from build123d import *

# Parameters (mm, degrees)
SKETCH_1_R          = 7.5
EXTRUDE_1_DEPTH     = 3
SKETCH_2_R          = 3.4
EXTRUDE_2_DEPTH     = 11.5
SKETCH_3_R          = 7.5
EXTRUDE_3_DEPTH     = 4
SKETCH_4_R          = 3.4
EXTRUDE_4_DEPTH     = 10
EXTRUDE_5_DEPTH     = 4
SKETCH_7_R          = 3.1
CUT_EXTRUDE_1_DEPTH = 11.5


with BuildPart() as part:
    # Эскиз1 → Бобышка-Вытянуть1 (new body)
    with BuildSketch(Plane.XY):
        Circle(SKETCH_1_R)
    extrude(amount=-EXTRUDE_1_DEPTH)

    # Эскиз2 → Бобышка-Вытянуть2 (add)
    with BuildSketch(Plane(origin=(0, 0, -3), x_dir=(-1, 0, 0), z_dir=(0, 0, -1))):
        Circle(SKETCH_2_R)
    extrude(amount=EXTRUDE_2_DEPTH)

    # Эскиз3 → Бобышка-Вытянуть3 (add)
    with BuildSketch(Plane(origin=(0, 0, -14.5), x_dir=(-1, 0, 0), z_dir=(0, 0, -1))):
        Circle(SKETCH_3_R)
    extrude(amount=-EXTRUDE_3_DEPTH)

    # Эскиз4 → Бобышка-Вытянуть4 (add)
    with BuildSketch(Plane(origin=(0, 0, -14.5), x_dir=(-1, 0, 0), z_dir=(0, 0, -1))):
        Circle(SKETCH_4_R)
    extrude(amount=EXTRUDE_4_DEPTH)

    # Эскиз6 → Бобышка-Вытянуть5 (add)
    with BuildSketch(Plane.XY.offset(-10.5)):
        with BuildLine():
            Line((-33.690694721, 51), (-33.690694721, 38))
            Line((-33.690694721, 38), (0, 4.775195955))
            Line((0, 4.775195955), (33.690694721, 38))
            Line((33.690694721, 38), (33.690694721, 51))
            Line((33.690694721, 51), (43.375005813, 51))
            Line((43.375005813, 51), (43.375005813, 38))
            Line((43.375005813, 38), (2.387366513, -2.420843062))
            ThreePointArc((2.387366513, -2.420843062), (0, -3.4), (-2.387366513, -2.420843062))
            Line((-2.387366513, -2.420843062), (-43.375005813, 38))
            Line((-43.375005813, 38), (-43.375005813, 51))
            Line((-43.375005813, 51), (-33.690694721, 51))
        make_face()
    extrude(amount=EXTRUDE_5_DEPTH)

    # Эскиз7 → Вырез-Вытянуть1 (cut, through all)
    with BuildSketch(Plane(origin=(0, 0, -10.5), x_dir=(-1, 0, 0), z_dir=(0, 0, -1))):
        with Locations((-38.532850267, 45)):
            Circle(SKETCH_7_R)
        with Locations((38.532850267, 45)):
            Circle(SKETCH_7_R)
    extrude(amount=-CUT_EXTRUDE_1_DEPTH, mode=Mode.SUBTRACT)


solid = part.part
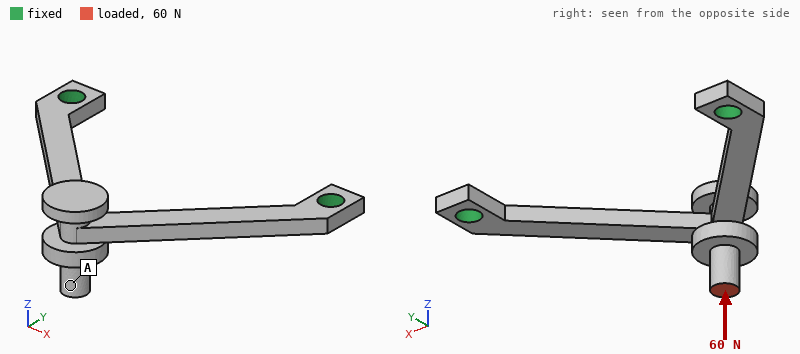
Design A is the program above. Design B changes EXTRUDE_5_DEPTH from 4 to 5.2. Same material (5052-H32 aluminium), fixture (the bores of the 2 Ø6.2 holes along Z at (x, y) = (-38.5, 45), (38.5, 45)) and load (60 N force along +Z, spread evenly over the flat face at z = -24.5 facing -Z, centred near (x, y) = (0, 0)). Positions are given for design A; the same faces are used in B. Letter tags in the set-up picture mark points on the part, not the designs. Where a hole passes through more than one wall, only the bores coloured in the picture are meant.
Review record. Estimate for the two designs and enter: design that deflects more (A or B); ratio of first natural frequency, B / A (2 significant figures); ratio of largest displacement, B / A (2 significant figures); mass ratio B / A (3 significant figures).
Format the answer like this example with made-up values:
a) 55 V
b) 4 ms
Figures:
a) A
b) 1.4
c) 0.49
d) 1.20
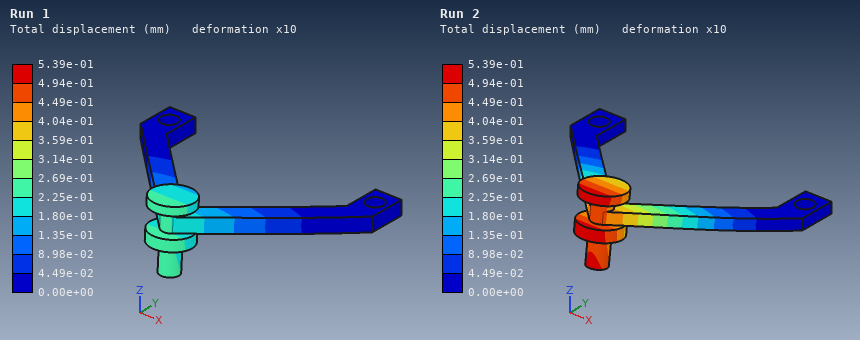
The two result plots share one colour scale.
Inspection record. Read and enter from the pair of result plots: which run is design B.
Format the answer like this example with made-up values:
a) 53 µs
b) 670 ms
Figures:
a) Run 1
